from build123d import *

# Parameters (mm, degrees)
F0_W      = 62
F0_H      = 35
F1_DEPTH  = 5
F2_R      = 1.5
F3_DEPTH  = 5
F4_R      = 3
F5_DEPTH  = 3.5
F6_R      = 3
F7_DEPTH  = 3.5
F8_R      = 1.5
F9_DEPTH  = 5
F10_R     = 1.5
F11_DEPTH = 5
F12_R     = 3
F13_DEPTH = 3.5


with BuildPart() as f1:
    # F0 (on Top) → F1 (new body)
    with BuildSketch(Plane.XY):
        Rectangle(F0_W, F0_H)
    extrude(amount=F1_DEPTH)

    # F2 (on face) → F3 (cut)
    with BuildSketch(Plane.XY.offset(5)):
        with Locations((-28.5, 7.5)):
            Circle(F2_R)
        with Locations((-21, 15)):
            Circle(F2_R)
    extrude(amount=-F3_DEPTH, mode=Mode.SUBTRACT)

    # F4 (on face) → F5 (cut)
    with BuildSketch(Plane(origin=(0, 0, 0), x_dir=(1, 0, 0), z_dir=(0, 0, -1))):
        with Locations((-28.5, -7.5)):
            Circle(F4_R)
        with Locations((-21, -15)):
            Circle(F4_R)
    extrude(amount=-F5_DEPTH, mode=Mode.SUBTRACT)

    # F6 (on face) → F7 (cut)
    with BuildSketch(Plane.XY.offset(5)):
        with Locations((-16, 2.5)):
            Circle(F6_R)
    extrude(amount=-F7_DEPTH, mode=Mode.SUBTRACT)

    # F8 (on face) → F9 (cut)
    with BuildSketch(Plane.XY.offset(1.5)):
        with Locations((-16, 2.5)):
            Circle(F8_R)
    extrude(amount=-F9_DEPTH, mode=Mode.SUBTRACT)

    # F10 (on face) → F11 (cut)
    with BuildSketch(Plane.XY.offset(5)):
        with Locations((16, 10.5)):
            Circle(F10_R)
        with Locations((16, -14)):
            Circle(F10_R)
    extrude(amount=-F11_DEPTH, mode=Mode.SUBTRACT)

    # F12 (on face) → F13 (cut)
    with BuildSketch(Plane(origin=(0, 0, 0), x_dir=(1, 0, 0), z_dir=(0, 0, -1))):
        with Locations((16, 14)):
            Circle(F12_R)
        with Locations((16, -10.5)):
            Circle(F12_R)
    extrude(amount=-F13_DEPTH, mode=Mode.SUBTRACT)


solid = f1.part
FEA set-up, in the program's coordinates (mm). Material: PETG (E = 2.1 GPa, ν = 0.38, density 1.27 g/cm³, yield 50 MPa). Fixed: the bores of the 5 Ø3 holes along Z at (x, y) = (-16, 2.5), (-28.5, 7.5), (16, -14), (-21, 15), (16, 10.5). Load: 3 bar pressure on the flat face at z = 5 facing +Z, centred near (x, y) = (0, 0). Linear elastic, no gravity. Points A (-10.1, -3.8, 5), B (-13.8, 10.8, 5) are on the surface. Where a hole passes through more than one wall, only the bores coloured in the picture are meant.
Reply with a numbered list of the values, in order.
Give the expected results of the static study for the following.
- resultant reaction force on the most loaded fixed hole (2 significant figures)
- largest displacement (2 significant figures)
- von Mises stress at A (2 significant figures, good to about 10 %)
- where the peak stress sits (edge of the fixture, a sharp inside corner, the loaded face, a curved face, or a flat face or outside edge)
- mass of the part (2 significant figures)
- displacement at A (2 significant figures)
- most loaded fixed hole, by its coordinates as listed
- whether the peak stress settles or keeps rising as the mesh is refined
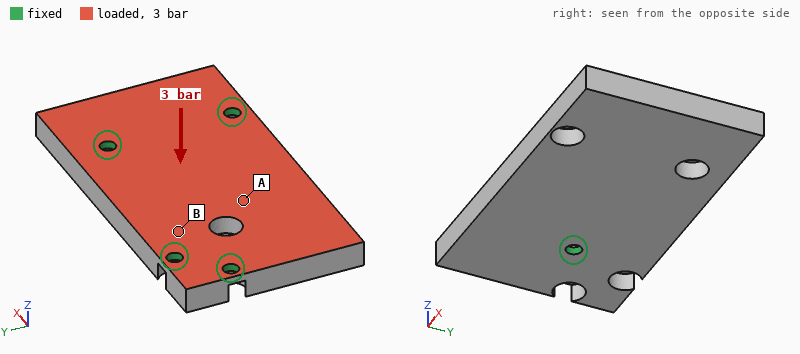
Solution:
1. 270 N
2. 0.55 mm
3. 7.7 MPa
4. edge of the fixture
5. 13 g
6. 0.16 mm
7. (-16, 2.5)
8. keeps rising
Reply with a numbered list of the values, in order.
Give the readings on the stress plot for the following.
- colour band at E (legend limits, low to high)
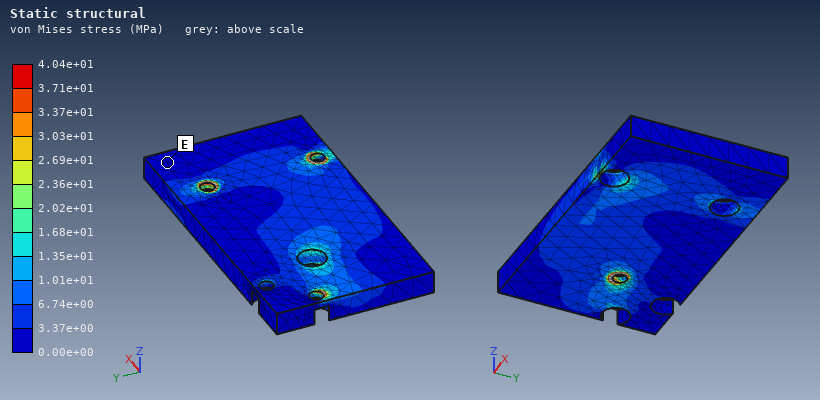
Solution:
1. 0.00e+00 to 3.37e+00 MPa
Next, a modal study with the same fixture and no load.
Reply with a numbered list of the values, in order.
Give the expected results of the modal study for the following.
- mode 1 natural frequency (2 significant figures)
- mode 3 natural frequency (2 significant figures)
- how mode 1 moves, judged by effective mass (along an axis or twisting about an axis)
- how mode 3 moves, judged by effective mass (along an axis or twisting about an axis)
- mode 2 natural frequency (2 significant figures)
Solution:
1. 1900 Hz
2. 3300 Hz
3. along Z
4. along Z
5. 2300 Hz
